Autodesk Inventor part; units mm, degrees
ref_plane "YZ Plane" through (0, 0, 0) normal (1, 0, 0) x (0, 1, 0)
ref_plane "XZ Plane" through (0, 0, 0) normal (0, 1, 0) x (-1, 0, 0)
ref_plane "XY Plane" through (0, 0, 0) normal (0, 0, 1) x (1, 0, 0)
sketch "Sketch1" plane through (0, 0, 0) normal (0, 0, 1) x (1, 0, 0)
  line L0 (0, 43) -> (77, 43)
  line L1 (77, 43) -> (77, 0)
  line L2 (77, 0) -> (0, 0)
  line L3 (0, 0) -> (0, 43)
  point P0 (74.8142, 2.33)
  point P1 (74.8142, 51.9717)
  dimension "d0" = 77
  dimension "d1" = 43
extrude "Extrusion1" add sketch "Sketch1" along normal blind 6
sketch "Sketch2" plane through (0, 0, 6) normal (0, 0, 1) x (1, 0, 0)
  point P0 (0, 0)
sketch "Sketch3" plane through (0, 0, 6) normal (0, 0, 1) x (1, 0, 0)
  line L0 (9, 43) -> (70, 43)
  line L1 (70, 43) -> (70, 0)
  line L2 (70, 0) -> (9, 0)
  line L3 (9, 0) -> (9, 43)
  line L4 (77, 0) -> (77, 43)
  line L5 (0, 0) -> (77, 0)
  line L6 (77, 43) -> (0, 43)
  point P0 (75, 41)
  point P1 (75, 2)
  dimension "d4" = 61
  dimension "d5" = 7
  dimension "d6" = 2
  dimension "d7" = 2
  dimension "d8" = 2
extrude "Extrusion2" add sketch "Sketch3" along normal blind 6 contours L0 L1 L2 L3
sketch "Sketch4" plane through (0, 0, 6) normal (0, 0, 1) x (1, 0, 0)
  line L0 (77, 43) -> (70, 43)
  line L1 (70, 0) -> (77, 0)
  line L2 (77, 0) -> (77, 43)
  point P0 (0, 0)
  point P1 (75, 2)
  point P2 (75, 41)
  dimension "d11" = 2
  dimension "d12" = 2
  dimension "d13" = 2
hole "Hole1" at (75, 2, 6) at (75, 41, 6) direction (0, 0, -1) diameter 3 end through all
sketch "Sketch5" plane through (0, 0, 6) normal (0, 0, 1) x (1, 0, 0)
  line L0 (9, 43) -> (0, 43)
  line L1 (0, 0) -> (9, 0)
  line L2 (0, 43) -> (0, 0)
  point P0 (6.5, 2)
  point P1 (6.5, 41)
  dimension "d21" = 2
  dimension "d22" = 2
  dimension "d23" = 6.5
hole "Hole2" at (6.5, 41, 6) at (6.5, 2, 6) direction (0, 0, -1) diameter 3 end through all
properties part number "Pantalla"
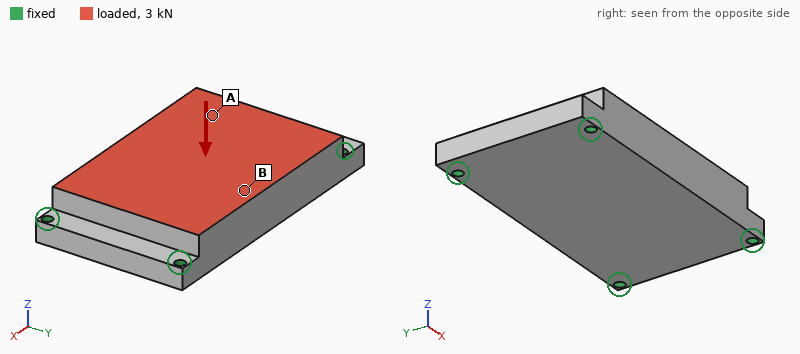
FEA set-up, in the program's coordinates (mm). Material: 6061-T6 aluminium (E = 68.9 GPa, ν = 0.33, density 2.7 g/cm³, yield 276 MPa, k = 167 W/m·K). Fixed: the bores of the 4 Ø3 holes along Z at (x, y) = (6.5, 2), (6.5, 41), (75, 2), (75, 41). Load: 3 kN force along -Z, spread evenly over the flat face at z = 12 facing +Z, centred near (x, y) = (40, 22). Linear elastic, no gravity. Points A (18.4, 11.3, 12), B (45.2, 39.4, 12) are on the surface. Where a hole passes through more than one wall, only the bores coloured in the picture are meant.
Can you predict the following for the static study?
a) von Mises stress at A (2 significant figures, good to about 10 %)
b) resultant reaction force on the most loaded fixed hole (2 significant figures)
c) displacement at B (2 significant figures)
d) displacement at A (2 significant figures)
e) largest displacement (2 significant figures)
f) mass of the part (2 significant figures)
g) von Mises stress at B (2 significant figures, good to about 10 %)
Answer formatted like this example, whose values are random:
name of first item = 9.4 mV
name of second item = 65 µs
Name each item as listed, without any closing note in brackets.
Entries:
von Mises stress at A = 9.0 MPa
resultant reaction force on the most loaded fixed hole = 1.0 kN
displacement at B = 23 µm
displacement at A = 14 µm
largest displacement = 24 µm
mass of the part = 96 g
von Mises stress at B = 19 MPa
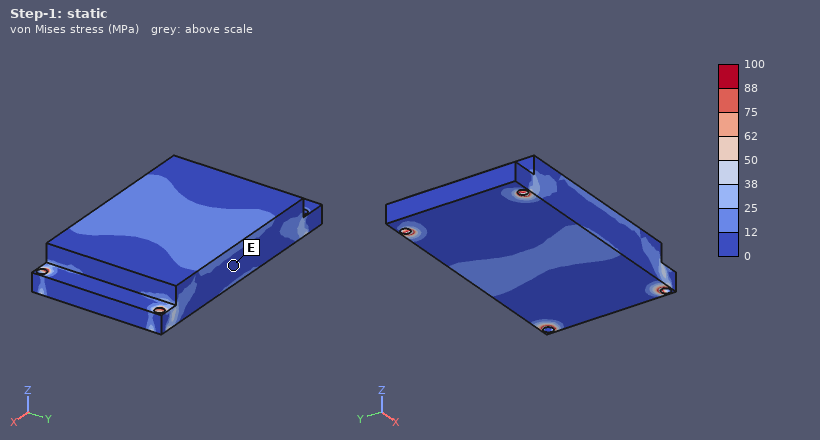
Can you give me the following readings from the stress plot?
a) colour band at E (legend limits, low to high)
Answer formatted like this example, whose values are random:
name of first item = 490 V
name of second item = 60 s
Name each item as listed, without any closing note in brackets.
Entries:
colour band at E = 0 to 12 MPa
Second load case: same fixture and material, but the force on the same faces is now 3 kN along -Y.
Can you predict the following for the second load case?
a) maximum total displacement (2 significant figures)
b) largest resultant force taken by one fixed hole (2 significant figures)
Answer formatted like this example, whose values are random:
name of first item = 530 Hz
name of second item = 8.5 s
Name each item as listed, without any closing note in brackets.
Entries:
maximum total displacement = 10 µm
largest resultant force taken by one fixed hole = 1.1 kN
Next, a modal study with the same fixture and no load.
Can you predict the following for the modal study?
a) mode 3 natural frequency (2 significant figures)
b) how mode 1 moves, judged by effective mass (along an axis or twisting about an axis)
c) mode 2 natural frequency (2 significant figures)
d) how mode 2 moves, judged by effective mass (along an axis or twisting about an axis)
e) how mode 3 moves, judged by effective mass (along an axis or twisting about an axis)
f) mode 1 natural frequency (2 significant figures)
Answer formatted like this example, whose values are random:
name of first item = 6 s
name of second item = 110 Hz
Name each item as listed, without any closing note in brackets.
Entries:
mode 3 natural frequency = 14 kHz
how mode 1 moves, judged by effective mass = along Z
mode 2 natural frequency = 11 kHz
how mode 2 moves, judged by effective mass = twisting about X
how mode 3 moves, judged by effective mass = along Y
mode 1 natural frequency = 6900 Hz
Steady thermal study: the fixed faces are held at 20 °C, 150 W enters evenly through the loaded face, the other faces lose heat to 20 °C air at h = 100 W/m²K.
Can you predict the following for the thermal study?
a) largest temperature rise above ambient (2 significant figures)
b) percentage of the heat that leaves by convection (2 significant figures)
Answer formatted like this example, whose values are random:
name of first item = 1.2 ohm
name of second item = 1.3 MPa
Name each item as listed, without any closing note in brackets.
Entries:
largest temperature rise above ambient = 35 K
percentage of the heat that leaves by convection = 10 %
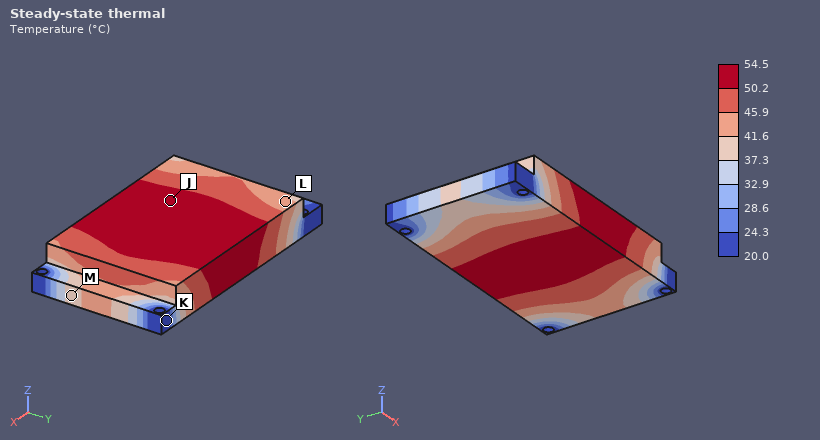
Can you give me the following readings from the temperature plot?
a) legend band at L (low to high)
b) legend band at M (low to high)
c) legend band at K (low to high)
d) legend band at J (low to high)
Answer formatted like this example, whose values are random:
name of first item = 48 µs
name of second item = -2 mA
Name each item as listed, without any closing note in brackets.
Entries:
legend band at L = 41.6 to 45.9 °C
legend band at M = 37.3 to 41.6 °C
legend band at K = 20.0 to 24.3 °C
legend band at J = 50.2 to 54.5 °C
